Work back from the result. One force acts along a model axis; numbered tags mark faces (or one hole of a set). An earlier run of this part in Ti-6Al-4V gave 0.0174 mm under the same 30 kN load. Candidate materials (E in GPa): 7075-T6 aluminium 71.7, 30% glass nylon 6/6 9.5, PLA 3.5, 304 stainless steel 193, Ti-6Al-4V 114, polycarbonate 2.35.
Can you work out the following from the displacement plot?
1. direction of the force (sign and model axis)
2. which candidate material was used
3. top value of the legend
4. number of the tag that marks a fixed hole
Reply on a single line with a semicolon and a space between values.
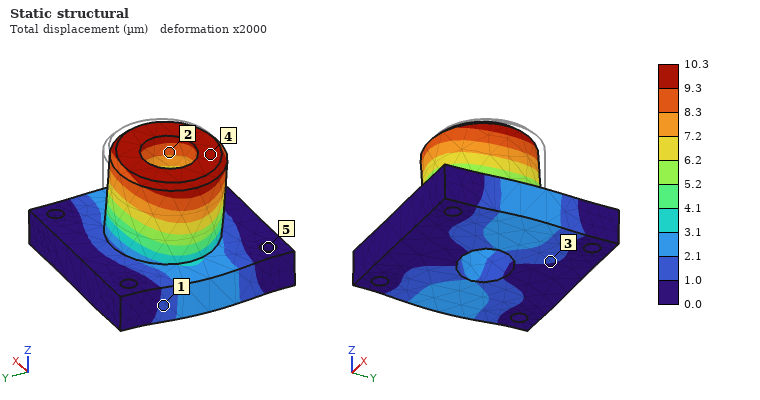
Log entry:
-X; 304 stainless steel; 10.3 µm; 5
